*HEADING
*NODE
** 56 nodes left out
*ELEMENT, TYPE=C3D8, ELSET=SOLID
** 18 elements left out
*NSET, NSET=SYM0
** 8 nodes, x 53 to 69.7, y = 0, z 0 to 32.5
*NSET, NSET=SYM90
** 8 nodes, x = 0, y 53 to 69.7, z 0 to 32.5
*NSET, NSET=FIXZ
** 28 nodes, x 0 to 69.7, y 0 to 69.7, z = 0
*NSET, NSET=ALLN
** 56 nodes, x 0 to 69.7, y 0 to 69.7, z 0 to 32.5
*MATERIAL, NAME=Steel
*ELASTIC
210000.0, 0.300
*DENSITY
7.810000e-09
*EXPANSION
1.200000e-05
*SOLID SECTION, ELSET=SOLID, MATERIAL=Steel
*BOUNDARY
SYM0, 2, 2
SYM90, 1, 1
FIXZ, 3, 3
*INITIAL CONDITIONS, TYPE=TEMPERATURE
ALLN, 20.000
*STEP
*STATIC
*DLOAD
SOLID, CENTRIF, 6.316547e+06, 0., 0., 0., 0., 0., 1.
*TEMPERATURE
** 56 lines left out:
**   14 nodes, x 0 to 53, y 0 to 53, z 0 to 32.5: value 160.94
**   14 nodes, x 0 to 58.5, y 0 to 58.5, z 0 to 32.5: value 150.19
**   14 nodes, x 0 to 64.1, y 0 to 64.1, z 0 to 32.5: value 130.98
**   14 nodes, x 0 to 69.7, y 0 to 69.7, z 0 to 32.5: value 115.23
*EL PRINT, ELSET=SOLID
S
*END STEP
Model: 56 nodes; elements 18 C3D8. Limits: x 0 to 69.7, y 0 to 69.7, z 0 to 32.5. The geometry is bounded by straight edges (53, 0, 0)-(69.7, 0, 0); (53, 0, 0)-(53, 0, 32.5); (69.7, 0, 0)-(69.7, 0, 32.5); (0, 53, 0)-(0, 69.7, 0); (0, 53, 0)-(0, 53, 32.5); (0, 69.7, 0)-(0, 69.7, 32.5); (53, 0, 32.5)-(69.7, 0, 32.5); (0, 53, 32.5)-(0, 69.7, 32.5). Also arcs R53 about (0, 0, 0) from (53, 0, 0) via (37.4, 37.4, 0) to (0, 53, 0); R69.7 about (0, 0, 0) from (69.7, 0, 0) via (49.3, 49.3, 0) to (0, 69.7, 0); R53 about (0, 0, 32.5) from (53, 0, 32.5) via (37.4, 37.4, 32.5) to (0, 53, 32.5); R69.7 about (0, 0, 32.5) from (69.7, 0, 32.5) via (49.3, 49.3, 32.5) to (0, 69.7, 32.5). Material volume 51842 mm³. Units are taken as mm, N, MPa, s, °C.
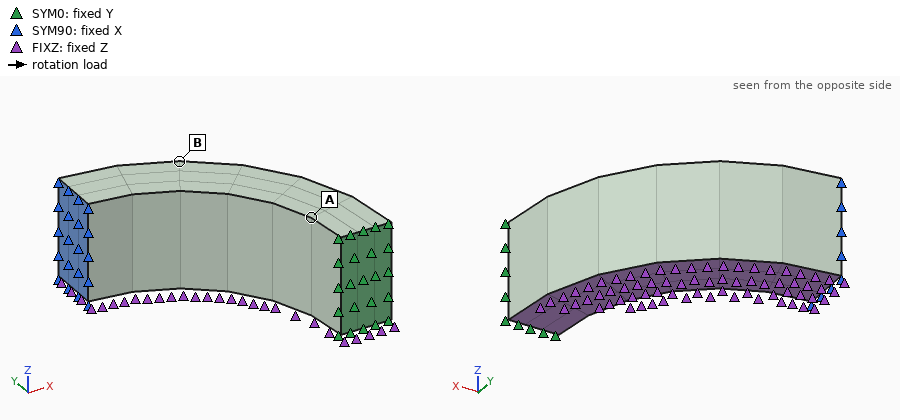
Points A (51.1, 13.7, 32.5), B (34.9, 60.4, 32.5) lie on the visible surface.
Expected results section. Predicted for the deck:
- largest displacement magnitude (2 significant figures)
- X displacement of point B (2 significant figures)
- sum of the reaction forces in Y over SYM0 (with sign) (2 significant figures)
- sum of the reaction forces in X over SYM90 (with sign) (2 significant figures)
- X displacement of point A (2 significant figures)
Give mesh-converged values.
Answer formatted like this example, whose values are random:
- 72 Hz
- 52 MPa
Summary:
- 0.16 mm
- 0.080 mm
- -100000 N
- -100000 N
- 0.14 mm
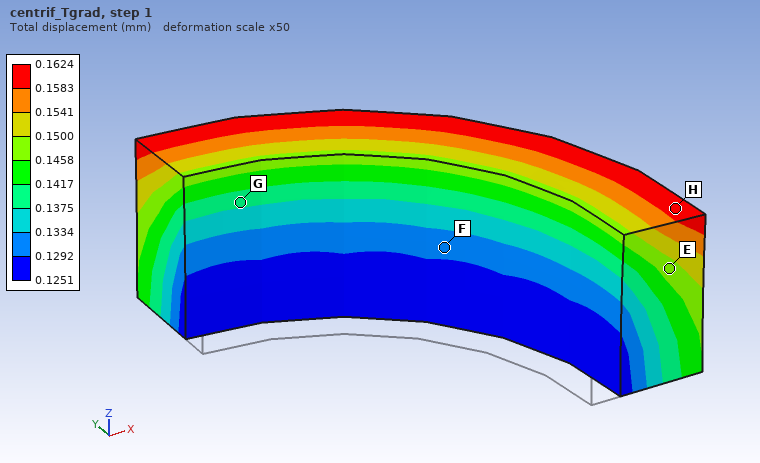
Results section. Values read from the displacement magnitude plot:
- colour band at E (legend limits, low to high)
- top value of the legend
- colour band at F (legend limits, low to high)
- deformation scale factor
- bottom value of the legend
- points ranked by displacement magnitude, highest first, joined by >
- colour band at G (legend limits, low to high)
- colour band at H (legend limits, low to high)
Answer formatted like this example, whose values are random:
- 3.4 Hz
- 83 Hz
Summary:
- 0.1458 to 0.1500 mm
- 0.1624 mm
- 0.1292 to 0.1334 mm
- 50
- 0.1251 mm
- H > E > G > F
- 0.1375 to 0.1417 mm
- 0.1583 to 0.1624 mm
